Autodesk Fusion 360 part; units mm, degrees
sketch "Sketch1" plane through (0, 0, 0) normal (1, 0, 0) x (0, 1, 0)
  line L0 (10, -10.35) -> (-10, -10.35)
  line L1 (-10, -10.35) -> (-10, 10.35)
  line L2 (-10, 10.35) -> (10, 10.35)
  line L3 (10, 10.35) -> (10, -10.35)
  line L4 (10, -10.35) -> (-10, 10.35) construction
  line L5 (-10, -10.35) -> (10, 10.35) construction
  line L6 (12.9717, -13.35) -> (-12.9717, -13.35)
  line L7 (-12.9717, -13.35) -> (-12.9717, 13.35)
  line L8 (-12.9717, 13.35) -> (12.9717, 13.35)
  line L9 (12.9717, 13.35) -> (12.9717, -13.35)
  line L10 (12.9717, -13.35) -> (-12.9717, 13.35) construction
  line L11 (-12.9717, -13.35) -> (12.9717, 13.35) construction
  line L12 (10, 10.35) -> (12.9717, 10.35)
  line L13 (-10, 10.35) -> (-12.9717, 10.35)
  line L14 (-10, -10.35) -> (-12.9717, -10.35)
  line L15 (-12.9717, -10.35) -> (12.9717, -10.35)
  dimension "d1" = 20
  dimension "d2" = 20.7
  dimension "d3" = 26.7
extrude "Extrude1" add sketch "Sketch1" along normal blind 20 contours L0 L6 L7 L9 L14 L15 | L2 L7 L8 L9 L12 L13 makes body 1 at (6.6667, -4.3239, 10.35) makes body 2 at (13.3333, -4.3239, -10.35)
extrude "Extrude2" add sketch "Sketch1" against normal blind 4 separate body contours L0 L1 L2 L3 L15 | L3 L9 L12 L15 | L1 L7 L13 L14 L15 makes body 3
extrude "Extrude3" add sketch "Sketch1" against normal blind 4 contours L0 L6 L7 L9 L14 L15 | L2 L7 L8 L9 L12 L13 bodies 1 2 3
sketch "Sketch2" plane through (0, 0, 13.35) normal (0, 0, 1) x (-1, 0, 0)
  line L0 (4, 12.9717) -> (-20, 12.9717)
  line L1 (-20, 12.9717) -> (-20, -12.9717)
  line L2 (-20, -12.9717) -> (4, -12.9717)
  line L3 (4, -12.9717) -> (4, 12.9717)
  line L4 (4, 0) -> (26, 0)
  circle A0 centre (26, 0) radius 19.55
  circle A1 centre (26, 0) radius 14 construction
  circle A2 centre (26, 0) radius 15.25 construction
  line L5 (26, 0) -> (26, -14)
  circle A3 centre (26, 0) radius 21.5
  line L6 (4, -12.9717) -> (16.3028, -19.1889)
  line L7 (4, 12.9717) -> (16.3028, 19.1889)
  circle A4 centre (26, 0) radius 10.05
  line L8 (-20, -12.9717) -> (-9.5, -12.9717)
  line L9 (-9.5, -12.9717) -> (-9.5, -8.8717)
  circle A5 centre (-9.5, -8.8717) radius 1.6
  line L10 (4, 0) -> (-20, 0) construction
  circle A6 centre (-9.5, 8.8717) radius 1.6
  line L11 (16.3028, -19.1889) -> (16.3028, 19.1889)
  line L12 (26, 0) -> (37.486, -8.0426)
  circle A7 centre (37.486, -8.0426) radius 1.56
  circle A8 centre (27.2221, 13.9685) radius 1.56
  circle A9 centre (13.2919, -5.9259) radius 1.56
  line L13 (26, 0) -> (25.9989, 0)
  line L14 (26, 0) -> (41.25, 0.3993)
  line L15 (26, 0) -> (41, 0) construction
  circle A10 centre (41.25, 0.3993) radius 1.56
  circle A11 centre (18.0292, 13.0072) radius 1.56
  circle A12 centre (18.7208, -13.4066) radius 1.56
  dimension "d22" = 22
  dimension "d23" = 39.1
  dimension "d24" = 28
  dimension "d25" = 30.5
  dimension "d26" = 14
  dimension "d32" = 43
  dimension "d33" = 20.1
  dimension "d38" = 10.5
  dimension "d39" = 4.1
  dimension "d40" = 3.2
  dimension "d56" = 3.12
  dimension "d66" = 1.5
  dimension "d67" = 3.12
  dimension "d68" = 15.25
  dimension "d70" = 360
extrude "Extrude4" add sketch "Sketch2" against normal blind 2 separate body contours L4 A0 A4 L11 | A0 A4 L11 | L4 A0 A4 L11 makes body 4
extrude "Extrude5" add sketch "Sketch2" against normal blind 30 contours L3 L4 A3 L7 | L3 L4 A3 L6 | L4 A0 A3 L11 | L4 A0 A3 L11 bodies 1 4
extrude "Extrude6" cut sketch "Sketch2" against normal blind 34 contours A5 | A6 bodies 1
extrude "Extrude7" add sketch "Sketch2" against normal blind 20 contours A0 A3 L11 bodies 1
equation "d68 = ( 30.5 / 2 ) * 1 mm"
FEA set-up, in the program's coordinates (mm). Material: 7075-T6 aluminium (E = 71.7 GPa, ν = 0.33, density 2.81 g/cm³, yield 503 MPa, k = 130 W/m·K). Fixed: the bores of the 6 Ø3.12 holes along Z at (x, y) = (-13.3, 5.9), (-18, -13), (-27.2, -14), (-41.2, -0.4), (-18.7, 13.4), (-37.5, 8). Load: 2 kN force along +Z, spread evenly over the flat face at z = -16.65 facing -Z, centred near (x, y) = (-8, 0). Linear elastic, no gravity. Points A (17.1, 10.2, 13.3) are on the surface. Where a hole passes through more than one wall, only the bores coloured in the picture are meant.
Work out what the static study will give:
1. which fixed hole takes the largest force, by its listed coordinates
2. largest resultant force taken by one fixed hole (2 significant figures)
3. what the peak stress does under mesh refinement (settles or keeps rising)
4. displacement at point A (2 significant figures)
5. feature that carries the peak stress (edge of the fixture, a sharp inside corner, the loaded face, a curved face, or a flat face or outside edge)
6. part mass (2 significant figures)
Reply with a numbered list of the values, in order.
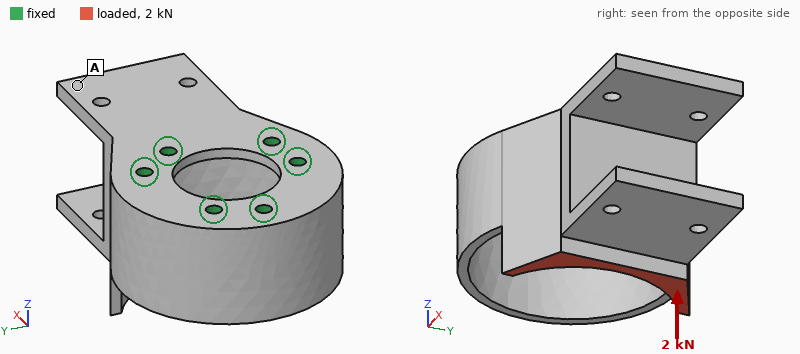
1. (-13.3, 5.9)
2. 1.1 kN
3. keeps rising
4. 0.14 mm
5. edge of the fixture
6. 44 g
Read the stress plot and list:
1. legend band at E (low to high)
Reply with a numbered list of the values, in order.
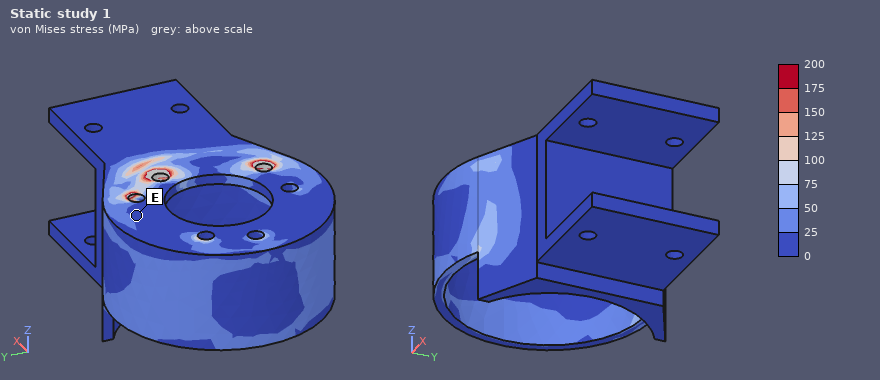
1. 0 to 25 MPa
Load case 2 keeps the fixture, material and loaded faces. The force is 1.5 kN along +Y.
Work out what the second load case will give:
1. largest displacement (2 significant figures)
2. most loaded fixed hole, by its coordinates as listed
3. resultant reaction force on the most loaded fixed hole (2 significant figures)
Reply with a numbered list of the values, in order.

1. 0.24 mm
2. (-18, -13)
3. 1.3 kN
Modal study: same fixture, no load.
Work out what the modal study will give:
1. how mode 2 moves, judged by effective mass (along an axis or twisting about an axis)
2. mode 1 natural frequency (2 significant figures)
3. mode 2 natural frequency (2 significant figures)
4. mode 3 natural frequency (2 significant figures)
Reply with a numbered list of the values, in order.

1. along Y
2. 2400 Hz
3. 4900 Hz
4. 5200 Hz
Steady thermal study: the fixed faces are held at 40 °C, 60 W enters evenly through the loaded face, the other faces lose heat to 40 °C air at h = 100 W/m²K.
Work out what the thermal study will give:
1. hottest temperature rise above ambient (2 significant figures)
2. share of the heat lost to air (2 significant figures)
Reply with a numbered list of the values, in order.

1. 67 K
2. 40 %
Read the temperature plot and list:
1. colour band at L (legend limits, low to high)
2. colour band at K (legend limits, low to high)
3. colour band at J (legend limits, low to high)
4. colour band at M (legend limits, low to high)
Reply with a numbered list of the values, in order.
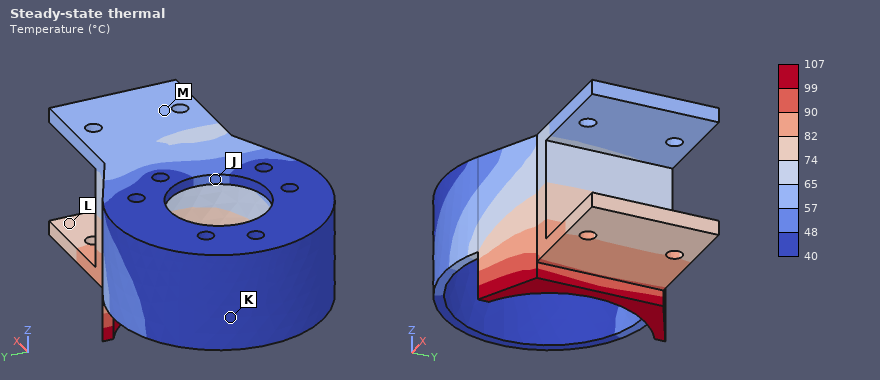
1. 74 to 82 °C
2. 40 to 48 °C
3. 48 to 57 °C
4. 57 to 65 °C
